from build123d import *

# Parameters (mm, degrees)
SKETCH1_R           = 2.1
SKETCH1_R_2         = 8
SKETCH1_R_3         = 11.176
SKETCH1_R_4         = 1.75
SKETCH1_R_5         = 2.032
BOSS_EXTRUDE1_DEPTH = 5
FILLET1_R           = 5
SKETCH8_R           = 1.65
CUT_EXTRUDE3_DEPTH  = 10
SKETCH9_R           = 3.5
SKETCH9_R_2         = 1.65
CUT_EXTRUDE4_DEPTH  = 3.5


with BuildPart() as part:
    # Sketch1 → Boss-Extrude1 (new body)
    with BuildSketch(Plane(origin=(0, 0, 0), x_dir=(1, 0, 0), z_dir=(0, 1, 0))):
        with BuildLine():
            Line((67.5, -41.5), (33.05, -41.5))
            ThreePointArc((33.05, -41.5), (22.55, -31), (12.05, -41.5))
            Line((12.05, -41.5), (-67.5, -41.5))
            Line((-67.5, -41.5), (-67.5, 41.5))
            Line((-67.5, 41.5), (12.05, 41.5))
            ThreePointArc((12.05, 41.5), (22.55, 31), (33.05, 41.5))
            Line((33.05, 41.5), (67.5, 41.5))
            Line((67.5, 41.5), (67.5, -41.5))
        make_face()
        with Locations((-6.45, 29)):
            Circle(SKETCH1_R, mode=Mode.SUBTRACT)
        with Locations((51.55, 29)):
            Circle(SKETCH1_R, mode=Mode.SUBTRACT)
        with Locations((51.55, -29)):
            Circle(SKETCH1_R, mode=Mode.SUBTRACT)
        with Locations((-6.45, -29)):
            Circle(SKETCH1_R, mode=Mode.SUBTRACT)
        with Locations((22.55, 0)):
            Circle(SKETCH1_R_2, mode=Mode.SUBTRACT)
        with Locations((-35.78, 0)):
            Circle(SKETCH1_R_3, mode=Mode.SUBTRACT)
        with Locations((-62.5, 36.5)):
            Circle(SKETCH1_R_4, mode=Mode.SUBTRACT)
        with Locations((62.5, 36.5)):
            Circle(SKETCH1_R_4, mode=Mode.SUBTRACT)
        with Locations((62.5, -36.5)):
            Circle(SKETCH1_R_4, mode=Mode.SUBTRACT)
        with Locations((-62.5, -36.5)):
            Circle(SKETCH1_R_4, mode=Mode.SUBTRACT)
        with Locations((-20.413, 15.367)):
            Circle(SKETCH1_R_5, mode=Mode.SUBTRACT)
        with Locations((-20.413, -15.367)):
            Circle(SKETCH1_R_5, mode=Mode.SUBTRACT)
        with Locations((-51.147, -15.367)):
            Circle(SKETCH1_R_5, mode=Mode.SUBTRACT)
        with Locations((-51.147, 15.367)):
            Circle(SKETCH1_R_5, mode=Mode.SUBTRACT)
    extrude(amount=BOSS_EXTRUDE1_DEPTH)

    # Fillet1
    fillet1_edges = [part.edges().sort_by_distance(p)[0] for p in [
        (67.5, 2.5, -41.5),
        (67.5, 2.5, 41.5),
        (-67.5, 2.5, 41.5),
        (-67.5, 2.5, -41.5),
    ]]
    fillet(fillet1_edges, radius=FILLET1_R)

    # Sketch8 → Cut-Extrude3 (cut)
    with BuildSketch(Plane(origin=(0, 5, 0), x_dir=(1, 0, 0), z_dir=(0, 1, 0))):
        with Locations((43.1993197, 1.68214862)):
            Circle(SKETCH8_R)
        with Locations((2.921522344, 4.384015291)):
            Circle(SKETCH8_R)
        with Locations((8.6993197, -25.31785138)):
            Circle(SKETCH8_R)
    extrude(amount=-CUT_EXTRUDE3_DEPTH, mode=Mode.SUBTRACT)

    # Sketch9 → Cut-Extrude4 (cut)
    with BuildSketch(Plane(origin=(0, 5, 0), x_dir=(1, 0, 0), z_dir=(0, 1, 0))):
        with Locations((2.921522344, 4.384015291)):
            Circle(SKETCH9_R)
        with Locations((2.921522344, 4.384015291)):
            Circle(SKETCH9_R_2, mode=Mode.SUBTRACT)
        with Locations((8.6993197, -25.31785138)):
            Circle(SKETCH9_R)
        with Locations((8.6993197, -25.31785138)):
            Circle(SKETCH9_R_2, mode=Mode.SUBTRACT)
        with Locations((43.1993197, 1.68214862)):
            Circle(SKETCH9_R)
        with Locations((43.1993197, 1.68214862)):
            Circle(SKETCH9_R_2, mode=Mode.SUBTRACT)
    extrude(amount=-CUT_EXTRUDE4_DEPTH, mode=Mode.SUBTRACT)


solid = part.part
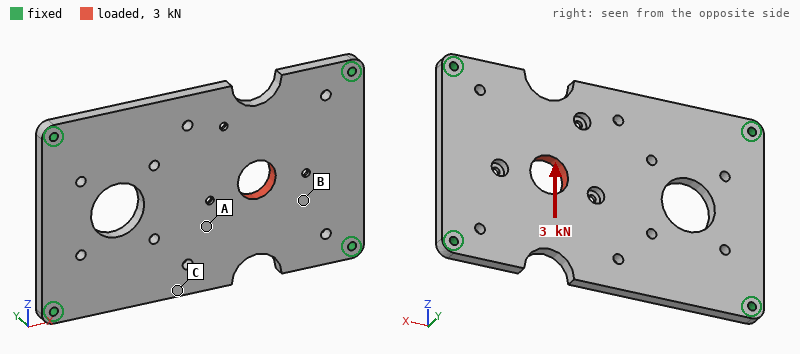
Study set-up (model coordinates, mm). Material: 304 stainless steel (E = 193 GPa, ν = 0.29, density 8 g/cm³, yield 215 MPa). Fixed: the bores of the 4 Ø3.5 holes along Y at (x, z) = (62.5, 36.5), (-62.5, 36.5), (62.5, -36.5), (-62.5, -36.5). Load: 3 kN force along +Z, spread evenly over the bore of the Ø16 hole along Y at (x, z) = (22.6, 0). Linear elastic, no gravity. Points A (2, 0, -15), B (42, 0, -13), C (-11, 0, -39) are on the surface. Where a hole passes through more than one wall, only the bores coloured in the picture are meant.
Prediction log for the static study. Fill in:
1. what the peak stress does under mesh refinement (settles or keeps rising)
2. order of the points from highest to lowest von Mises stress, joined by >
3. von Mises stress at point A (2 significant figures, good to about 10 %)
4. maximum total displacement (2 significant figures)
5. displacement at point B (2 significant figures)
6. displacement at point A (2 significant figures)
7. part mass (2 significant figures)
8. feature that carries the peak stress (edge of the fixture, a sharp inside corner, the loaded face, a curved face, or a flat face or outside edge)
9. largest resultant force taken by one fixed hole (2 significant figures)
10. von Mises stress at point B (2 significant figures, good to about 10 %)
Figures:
keeps rising
B > A > C
6.8 MPa
5.8 µm
3.1 µm
4.5 µm
400 g
edge of the fixture
1.3 kN
14 MPa
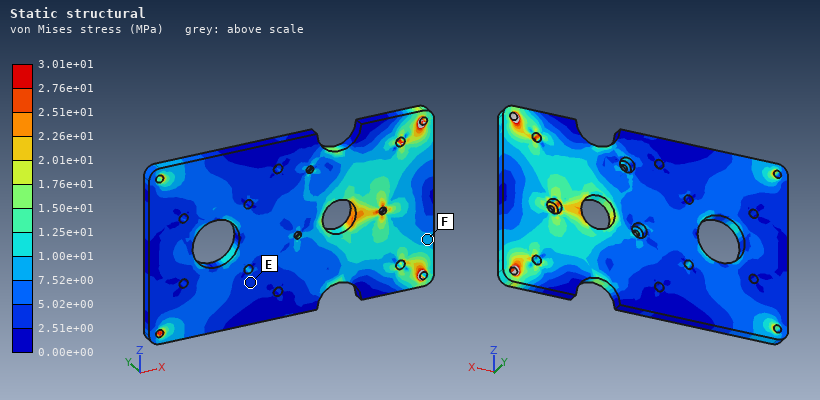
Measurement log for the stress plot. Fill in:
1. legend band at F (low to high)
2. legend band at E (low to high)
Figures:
7.52e+00 to 1.00e+01 MPa
2.51e+00 to 5.02e+00 MPa
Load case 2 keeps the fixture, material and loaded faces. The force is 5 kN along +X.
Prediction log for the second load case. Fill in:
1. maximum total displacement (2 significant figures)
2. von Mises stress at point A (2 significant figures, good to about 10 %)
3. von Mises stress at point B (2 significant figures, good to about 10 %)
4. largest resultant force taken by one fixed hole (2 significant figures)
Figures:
5.8 µm
11 MPa
12 MPa
1.6 kN
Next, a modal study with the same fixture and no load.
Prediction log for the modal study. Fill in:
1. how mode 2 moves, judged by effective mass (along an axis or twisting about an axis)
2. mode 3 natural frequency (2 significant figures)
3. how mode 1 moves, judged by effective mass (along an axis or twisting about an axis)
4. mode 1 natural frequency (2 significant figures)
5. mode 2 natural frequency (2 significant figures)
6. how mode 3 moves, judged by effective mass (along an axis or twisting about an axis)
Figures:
twisting about X
3200 Hz
along Y
1200 Hz
2100 Hz
twisting about Z
